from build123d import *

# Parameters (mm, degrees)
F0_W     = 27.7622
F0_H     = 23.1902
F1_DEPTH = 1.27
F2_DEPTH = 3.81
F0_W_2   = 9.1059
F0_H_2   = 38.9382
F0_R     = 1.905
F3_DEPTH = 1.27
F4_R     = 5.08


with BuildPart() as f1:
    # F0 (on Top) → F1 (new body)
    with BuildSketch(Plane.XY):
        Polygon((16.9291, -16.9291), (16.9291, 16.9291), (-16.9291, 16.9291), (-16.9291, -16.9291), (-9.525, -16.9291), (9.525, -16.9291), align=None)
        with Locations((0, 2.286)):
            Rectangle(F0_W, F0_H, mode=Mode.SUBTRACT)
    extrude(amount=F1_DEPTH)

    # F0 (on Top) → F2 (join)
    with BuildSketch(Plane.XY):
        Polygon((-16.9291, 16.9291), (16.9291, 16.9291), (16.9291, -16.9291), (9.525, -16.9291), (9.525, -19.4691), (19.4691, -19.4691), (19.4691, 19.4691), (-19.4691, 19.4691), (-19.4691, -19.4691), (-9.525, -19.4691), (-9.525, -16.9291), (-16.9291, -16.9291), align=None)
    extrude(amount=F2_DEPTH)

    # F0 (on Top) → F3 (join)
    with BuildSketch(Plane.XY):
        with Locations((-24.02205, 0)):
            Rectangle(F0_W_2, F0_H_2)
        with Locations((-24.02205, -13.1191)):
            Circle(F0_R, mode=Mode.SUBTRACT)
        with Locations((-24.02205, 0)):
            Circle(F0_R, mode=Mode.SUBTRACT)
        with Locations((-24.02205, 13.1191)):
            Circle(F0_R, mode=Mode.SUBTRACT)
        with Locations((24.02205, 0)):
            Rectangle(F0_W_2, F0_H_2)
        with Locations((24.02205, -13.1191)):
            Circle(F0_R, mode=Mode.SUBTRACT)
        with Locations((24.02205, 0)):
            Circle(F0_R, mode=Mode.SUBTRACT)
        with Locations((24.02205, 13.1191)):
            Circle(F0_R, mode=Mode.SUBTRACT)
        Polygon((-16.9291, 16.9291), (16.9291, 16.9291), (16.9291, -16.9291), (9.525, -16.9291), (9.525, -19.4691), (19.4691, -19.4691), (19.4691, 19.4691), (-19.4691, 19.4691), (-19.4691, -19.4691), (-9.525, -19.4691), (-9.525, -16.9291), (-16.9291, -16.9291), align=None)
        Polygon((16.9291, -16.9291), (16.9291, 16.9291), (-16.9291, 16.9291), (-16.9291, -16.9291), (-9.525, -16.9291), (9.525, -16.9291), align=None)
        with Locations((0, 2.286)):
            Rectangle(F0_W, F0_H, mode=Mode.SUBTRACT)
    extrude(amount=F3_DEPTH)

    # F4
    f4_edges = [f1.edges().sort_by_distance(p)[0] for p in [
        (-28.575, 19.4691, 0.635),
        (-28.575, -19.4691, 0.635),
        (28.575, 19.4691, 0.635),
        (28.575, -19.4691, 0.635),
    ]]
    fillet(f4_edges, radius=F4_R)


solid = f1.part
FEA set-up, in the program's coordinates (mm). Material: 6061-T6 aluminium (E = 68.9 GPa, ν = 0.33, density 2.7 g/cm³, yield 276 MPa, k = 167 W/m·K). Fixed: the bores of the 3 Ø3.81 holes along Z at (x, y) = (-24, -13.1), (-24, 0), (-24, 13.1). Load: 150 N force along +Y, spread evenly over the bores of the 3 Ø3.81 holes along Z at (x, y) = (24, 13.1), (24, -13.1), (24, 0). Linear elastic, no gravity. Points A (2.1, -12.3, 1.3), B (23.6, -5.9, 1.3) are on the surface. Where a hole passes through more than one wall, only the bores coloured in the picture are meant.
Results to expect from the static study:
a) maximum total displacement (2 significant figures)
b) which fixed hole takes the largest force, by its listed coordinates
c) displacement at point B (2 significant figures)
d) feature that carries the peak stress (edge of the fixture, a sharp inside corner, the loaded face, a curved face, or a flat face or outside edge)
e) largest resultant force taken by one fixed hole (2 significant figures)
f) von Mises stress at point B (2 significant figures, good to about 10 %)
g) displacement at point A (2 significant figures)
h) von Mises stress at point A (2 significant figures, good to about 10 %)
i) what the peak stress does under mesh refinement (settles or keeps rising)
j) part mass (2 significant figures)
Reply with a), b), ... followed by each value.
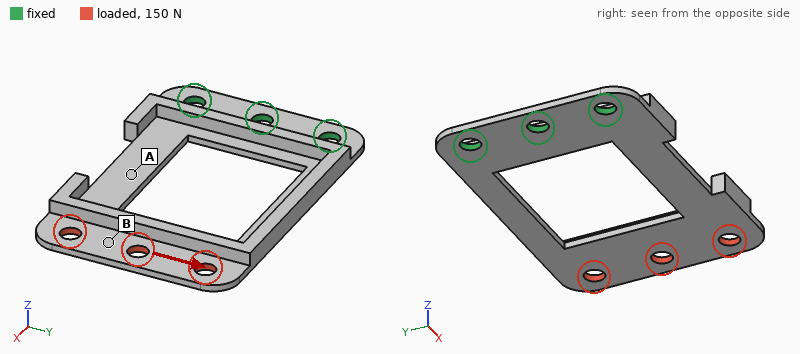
a) 0.16 mm
b) (-24, -13.1)
c) 0.15 mm
d) a sharp inside corner
e) 260 N
f) 12 MPa
g) 0.066 mm
h) 34 MPa
i) keeps rising
j) 7.2 g
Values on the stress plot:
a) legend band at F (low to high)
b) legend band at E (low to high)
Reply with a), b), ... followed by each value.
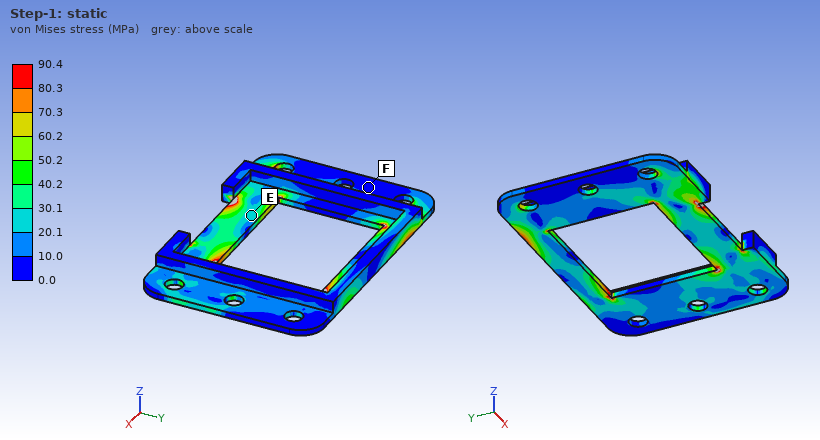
a) 0.0 to 10.0 MPa
b) 20.1 to 30.1 MPa
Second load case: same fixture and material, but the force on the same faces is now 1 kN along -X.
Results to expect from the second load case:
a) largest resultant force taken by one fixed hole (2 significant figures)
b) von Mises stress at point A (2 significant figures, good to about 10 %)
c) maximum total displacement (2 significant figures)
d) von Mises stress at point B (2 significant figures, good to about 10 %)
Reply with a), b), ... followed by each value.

a) 500 N
b) 49 MPa
c) 0.30 mm
d) 26 MPa
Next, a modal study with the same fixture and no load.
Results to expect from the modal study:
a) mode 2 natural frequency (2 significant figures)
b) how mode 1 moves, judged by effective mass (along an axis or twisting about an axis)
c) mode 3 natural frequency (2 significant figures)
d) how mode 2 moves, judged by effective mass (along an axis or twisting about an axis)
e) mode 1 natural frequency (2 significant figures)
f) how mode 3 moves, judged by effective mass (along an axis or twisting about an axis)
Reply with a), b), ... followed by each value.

a) 1200 Hz
b) along Z
c) 3200 Hz
d) twisting about X
e) 450 Hz
f) along Y
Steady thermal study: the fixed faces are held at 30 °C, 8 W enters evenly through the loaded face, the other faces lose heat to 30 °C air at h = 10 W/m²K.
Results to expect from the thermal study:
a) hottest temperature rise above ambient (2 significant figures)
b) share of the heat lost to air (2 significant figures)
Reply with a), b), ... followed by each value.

a) 74 K
b) 17 %
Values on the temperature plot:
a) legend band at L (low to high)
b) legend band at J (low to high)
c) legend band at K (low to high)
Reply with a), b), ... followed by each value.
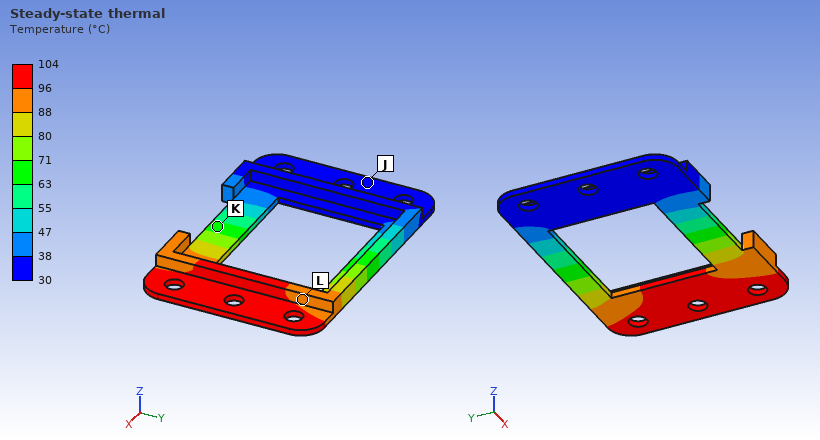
a) 88 to 96 °C
b) 30 to 38 °C
c) 63 to 71 °C
